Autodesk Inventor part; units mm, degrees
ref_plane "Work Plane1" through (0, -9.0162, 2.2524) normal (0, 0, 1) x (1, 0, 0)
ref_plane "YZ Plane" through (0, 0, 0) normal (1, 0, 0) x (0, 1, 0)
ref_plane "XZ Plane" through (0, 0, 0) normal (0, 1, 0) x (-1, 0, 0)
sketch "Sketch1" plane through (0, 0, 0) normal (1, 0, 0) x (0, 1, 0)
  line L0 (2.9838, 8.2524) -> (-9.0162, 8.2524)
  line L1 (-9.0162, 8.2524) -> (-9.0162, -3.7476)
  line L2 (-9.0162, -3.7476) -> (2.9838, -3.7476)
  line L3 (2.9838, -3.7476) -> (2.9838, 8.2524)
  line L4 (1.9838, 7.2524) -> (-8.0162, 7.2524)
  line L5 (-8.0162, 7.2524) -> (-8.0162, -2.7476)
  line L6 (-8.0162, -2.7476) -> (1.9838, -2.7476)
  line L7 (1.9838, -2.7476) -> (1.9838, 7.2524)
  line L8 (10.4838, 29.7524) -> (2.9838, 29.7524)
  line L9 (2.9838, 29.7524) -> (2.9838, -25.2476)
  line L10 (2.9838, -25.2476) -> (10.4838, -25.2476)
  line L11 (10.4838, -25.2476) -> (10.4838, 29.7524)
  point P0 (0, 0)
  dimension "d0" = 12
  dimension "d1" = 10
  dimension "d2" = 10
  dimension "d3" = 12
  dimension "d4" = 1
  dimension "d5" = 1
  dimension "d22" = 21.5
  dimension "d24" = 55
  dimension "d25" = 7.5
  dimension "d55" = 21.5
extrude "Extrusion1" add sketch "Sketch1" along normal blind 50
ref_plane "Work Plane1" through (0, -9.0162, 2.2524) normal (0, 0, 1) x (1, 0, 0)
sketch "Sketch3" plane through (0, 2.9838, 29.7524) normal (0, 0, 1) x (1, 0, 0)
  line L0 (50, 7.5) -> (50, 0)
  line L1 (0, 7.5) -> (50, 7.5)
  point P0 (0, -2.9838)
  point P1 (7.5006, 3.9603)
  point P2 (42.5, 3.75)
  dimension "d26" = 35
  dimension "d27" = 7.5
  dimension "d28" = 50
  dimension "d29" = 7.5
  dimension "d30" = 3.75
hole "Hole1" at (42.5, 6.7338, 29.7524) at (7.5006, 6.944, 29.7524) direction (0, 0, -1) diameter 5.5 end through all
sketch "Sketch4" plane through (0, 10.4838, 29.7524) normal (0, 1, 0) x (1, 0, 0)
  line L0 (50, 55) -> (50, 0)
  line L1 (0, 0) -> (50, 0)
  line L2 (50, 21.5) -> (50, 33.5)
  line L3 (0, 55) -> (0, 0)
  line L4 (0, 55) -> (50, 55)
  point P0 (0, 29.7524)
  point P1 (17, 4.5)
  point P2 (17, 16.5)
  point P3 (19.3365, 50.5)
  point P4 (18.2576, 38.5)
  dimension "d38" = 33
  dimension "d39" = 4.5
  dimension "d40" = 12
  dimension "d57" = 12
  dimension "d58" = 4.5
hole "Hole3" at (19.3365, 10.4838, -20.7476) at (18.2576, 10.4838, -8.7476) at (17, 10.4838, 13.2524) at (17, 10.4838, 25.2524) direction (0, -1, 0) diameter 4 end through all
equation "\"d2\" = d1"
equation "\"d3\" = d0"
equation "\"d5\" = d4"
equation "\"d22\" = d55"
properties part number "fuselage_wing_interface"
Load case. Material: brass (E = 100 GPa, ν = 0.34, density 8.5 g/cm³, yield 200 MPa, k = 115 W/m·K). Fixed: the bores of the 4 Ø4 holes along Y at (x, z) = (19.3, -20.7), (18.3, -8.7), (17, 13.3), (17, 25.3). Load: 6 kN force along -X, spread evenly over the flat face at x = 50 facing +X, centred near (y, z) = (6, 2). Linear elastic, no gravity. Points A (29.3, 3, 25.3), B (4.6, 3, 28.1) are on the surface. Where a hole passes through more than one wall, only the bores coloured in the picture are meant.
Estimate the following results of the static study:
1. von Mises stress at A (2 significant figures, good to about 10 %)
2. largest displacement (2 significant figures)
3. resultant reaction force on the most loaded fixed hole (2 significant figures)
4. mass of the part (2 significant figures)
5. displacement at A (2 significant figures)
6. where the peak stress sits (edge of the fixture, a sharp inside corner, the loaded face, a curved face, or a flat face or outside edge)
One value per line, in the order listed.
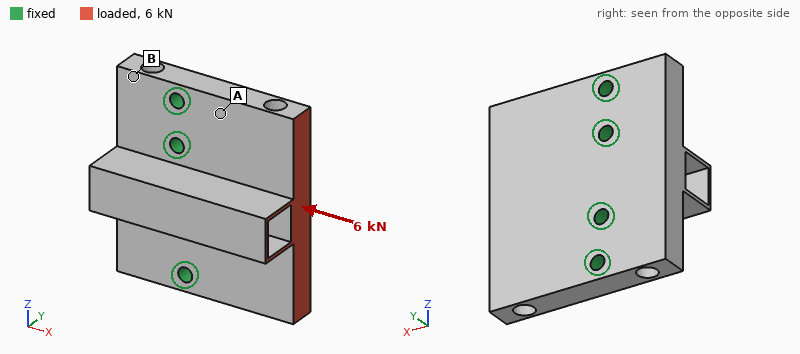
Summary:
17 MPa
11 µm
1.7 kN
170 g
2.7 µm
a curved face
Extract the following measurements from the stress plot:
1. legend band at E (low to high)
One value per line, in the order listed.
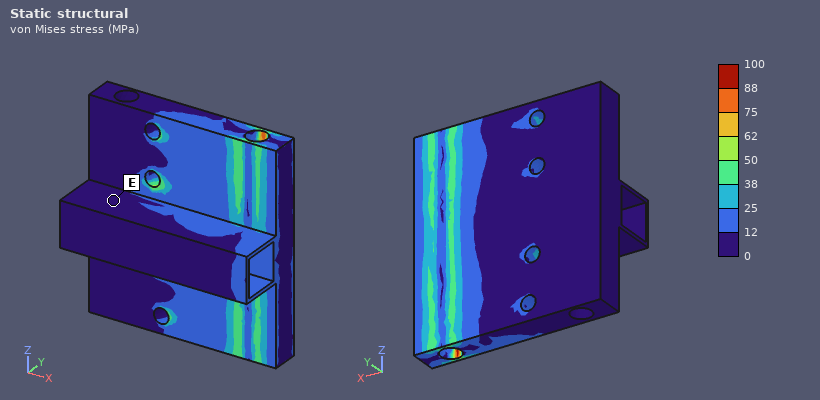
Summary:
0 to 12 MPa
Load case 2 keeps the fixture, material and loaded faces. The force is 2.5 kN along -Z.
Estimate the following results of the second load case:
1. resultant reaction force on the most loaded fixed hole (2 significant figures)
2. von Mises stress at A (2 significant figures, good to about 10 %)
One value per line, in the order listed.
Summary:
1.6 kN
13 MPa
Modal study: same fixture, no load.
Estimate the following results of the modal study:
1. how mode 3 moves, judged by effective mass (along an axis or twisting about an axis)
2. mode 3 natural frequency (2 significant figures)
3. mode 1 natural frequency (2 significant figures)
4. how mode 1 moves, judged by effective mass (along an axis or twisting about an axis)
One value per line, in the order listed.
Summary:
twisting about X
7200 Hz
4400 Hz
along Y
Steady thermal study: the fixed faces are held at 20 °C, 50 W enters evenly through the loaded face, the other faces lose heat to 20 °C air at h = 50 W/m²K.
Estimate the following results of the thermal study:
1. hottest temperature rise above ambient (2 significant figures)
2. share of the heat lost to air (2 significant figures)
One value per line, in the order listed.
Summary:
39 K
13 %
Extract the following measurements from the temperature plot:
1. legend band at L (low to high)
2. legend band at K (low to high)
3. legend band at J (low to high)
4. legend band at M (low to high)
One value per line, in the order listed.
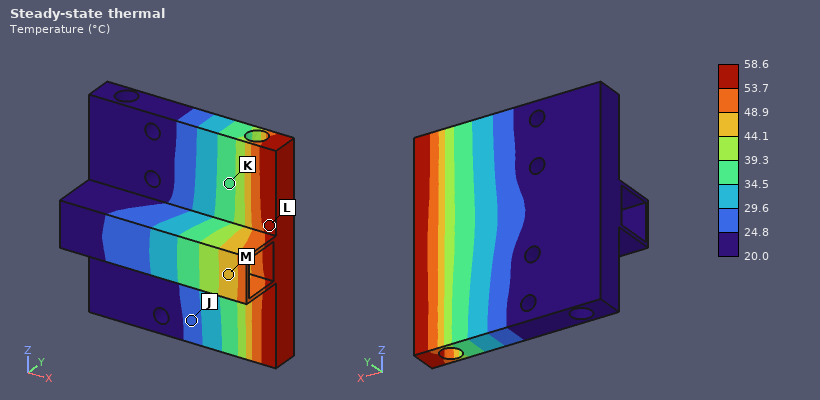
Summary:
53.7 to 58.6 °C
34.5 to 39.3 °C
24.8 to 29.6 °C
44.1 to 48.9 °C
